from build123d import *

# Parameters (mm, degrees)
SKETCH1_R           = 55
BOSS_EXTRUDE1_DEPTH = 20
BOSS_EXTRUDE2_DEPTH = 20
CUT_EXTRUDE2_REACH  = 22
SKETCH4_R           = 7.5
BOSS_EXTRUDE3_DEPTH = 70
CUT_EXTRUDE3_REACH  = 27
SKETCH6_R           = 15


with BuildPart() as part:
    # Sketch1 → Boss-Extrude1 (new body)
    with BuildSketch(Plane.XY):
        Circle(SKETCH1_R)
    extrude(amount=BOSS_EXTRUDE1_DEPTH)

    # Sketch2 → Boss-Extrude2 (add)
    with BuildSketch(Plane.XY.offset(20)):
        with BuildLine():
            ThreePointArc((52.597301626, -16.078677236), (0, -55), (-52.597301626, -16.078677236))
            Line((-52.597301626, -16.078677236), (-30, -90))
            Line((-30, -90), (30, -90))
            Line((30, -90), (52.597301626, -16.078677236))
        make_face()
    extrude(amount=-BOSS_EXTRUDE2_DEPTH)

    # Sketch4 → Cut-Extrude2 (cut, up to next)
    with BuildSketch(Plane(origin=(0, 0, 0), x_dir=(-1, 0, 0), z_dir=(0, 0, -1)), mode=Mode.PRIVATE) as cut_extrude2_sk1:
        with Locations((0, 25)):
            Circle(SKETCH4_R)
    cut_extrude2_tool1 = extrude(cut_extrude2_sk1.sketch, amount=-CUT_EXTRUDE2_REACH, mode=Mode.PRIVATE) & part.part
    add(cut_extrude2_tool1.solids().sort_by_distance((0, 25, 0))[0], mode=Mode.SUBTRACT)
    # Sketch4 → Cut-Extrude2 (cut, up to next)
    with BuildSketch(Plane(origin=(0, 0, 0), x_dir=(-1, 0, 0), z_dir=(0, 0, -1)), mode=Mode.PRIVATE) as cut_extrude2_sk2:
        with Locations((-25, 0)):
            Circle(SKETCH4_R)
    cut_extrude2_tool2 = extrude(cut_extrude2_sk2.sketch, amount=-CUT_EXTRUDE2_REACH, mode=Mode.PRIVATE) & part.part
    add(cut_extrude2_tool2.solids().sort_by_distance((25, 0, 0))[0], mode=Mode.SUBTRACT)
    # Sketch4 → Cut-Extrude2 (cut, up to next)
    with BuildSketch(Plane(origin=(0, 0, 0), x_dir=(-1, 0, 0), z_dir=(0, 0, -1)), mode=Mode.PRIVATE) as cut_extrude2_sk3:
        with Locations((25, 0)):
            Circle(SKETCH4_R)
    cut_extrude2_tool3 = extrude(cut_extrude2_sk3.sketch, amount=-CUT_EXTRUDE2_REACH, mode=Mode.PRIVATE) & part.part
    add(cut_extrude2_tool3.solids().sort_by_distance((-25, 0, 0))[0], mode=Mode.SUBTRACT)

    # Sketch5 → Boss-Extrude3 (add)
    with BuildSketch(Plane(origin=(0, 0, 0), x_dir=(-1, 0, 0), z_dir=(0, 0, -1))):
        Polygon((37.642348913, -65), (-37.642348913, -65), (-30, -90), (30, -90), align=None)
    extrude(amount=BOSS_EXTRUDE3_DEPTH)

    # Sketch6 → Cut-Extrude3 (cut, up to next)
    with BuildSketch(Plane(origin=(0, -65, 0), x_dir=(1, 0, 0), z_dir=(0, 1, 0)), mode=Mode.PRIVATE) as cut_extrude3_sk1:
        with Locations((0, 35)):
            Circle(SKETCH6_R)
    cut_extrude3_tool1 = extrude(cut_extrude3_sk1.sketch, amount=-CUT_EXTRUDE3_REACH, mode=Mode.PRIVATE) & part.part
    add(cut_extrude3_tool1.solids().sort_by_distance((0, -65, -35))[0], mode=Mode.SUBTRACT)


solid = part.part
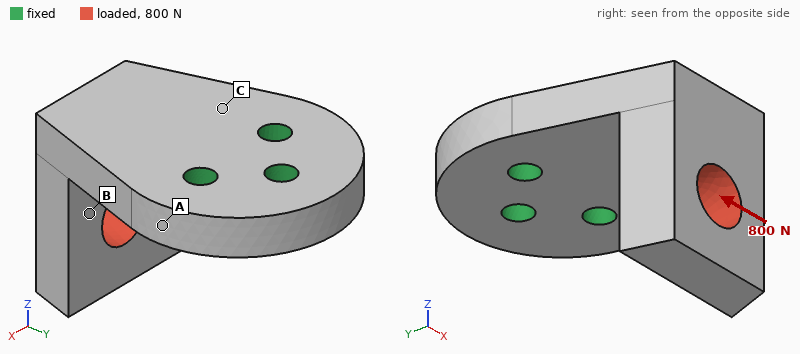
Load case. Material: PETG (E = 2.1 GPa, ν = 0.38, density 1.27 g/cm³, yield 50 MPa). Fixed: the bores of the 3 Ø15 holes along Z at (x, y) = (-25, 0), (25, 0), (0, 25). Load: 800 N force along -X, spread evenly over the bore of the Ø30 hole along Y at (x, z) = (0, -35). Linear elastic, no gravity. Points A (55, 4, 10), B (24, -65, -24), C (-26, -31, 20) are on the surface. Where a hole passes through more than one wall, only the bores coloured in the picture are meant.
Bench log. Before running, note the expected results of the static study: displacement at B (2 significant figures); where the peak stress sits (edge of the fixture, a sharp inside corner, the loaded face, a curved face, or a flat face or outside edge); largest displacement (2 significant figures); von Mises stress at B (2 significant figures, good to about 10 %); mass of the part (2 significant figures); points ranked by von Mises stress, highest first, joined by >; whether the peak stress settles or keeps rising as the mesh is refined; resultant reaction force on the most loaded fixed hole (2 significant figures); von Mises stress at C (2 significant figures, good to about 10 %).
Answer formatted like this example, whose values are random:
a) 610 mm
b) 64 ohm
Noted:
a) 0.49 mm
b) edge of the fixture
c) 1.0 mm
d) 1.9 MPa
e) 430 g
f) C > B > A
g) keeps rising
h) 1.2 kN
i) 3.2 MPa
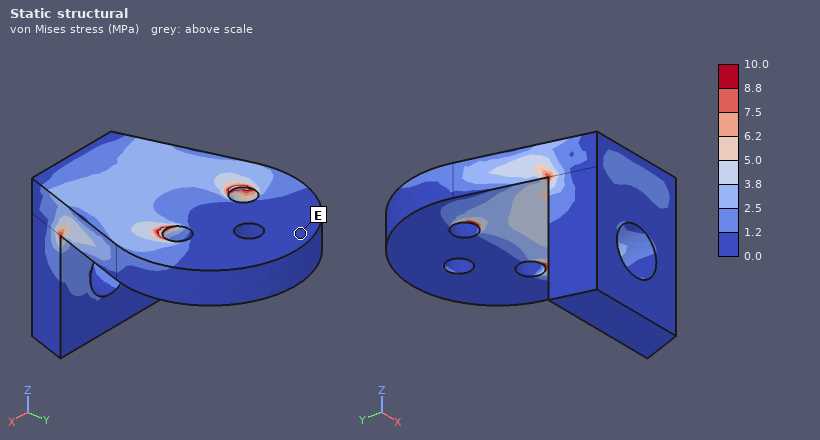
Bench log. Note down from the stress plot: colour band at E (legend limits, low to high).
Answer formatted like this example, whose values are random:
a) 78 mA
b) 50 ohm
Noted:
a) 0.0 to 1.2 MPa
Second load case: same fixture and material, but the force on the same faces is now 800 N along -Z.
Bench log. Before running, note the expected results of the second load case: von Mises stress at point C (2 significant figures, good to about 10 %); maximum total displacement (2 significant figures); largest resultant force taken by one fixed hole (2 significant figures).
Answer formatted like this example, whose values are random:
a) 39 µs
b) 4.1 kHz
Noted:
a) 5.7 MPa
b) 1.7 mm
c) 520 N
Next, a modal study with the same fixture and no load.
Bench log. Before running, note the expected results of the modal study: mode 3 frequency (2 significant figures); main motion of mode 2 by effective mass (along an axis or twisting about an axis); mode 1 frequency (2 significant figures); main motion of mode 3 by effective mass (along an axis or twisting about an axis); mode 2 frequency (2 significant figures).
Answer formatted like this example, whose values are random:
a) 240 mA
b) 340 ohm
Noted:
a) 720 Hz
b) along X
c) 260 Hz
d) along Z
e) 450 Hz
